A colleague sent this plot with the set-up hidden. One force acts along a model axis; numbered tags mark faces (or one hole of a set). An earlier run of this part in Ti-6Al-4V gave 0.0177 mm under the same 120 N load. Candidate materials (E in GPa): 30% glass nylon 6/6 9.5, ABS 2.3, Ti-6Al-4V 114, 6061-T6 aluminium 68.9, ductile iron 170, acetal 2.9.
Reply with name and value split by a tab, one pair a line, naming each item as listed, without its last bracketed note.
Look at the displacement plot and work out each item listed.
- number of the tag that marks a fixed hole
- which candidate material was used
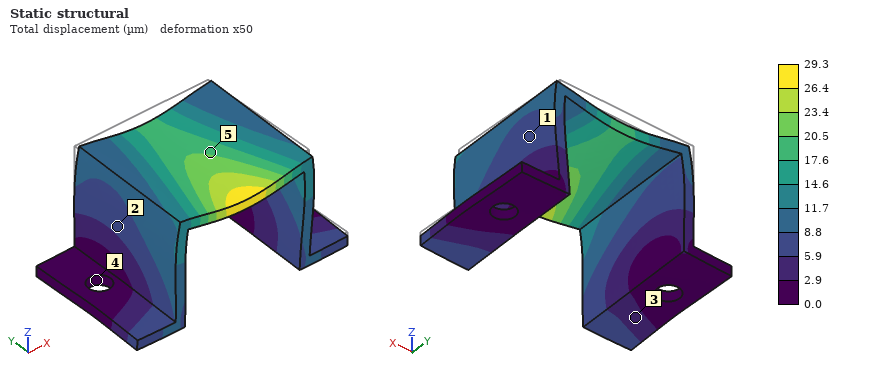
number of the tag that marks a fixed hole	4
which candidate material was used	6061-T6 aluminium
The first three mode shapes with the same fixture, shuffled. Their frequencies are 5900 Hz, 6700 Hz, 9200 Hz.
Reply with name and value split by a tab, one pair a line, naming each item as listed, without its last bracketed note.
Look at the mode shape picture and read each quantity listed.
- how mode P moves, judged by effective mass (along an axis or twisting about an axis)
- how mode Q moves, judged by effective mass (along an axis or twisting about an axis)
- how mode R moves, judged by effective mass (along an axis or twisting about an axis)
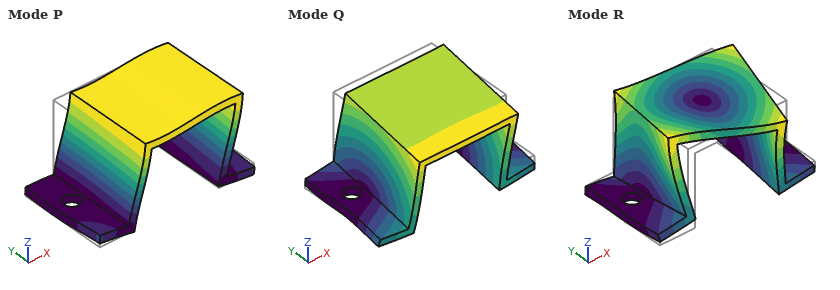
how mode P moves, judged by effective mass	along X
how mode Q moves, judged by effective mass	along Y
how mode R moves, judged by effective mass	twisting about Z
